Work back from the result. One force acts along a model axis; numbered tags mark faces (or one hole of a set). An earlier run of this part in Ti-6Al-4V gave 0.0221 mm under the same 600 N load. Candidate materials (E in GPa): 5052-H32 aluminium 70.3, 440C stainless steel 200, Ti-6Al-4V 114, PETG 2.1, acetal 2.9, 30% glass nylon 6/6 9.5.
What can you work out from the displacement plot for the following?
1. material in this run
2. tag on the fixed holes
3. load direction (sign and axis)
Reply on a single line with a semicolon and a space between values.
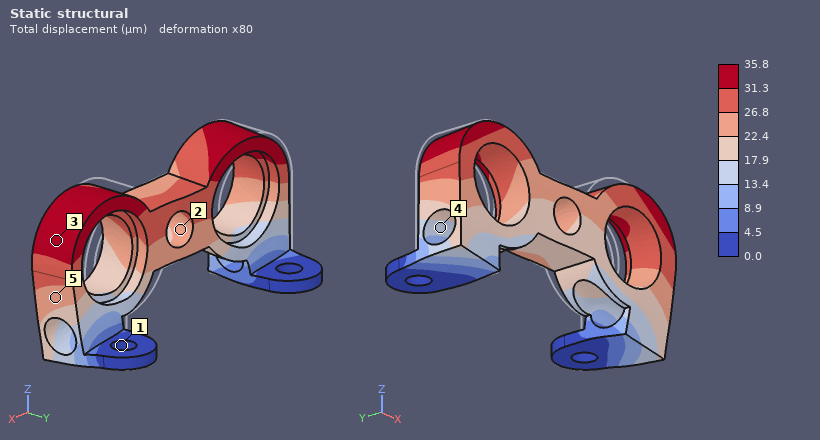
5052-H32 aluminium; 1; +X
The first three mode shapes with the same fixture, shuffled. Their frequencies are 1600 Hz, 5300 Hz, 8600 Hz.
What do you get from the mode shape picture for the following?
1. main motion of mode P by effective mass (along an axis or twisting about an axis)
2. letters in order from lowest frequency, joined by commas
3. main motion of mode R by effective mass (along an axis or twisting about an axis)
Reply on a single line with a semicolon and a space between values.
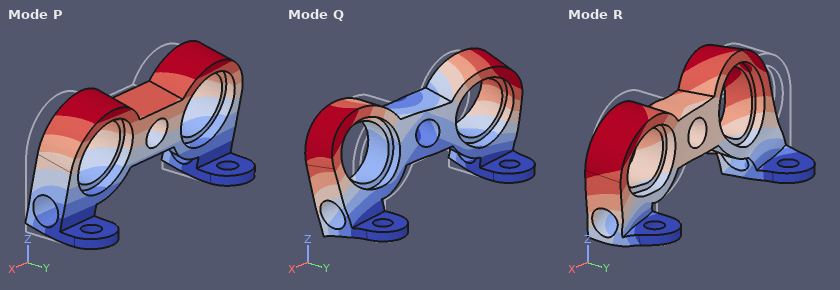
along Y; P, Q, R; along X
